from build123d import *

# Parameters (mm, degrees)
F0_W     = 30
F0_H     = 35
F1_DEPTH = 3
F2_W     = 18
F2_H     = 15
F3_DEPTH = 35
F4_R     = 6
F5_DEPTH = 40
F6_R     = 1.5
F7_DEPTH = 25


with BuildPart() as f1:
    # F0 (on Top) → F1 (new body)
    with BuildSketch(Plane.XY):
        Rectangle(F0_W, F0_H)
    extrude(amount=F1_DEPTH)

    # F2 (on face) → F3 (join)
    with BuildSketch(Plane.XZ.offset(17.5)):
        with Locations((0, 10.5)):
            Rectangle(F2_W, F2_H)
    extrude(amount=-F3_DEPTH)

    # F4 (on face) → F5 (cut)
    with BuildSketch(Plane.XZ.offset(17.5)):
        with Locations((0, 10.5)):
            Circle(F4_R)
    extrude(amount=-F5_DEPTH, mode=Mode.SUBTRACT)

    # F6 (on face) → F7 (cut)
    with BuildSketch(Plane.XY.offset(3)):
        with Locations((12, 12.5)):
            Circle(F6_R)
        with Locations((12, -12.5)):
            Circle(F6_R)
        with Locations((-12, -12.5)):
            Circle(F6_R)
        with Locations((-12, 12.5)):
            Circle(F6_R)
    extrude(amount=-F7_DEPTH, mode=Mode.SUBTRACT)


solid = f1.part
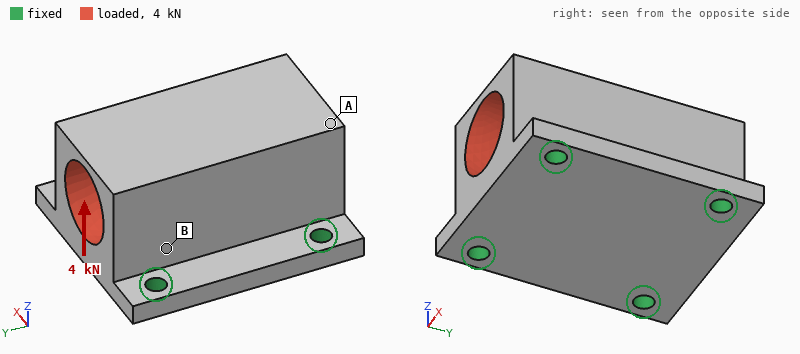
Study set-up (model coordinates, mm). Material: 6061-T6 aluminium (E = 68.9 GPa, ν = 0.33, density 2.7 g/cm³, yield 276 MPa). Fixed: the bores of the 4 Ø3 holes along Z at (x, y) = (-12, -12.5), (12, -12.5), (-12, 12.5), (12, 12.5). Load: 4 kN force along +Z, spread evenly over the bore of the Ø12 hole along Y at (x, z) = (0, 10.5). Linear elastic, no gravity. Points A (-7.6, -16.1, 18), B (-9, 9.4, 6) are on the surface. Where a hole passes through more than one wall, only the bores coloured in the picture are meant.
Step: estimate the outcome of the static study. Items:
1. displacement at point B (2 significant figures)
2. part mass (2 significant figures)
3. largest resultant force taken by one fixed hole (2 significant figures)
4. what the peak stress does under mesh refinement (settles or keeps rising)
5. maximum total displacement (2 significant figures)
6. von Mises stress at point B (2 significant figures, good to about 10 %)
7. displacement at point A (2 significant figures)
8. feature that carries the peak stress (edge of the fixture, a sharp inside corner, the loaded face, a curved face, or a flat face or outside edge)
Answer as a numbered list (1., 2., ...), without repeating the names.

1. 11 µm
2. 23 g
3. 1.1 kN
4. keeps rising
5. 15 µm
6. 39 MPa
7. 11 µm
8. edge of the fixture
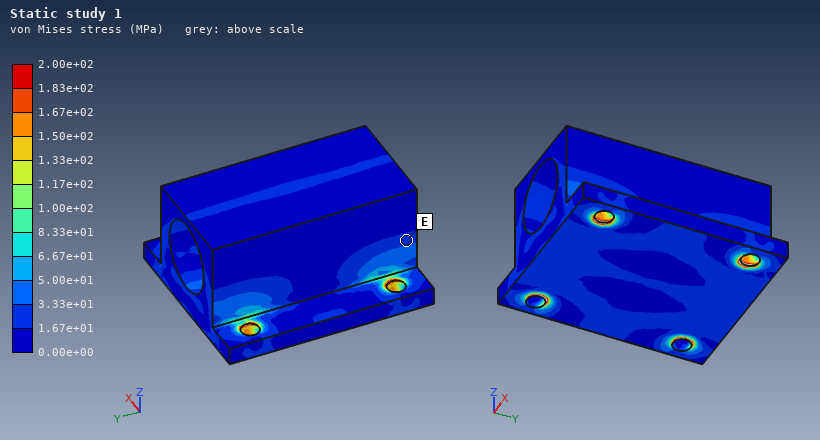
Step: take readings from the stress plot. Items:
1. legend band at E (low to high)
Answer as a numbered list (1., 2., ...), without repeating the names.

1. 1.67e+01 to 3.33e+01 MPa
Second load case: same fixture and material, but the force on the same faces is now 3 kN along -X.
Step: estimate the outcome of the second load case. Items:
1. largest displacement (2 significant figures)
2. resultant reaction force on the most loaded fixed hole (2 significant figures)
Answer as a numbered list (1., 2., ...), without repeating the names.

1. 30 µm
2. 1.0 kN
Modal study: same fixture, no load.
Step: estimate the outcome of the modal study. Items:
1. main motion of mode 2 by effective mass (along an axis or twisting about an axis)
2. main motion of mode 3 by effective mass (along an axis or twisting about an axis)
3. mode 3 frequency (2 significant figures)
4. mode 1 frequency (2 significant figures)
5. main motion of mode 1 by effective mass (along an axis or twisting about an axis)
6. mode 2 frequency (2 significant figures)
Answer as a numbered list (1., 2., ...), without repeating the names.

1. along Y
2. along Z
3. 19 kHz
4. 15 kHz
5. along X
6. 17 kHz
